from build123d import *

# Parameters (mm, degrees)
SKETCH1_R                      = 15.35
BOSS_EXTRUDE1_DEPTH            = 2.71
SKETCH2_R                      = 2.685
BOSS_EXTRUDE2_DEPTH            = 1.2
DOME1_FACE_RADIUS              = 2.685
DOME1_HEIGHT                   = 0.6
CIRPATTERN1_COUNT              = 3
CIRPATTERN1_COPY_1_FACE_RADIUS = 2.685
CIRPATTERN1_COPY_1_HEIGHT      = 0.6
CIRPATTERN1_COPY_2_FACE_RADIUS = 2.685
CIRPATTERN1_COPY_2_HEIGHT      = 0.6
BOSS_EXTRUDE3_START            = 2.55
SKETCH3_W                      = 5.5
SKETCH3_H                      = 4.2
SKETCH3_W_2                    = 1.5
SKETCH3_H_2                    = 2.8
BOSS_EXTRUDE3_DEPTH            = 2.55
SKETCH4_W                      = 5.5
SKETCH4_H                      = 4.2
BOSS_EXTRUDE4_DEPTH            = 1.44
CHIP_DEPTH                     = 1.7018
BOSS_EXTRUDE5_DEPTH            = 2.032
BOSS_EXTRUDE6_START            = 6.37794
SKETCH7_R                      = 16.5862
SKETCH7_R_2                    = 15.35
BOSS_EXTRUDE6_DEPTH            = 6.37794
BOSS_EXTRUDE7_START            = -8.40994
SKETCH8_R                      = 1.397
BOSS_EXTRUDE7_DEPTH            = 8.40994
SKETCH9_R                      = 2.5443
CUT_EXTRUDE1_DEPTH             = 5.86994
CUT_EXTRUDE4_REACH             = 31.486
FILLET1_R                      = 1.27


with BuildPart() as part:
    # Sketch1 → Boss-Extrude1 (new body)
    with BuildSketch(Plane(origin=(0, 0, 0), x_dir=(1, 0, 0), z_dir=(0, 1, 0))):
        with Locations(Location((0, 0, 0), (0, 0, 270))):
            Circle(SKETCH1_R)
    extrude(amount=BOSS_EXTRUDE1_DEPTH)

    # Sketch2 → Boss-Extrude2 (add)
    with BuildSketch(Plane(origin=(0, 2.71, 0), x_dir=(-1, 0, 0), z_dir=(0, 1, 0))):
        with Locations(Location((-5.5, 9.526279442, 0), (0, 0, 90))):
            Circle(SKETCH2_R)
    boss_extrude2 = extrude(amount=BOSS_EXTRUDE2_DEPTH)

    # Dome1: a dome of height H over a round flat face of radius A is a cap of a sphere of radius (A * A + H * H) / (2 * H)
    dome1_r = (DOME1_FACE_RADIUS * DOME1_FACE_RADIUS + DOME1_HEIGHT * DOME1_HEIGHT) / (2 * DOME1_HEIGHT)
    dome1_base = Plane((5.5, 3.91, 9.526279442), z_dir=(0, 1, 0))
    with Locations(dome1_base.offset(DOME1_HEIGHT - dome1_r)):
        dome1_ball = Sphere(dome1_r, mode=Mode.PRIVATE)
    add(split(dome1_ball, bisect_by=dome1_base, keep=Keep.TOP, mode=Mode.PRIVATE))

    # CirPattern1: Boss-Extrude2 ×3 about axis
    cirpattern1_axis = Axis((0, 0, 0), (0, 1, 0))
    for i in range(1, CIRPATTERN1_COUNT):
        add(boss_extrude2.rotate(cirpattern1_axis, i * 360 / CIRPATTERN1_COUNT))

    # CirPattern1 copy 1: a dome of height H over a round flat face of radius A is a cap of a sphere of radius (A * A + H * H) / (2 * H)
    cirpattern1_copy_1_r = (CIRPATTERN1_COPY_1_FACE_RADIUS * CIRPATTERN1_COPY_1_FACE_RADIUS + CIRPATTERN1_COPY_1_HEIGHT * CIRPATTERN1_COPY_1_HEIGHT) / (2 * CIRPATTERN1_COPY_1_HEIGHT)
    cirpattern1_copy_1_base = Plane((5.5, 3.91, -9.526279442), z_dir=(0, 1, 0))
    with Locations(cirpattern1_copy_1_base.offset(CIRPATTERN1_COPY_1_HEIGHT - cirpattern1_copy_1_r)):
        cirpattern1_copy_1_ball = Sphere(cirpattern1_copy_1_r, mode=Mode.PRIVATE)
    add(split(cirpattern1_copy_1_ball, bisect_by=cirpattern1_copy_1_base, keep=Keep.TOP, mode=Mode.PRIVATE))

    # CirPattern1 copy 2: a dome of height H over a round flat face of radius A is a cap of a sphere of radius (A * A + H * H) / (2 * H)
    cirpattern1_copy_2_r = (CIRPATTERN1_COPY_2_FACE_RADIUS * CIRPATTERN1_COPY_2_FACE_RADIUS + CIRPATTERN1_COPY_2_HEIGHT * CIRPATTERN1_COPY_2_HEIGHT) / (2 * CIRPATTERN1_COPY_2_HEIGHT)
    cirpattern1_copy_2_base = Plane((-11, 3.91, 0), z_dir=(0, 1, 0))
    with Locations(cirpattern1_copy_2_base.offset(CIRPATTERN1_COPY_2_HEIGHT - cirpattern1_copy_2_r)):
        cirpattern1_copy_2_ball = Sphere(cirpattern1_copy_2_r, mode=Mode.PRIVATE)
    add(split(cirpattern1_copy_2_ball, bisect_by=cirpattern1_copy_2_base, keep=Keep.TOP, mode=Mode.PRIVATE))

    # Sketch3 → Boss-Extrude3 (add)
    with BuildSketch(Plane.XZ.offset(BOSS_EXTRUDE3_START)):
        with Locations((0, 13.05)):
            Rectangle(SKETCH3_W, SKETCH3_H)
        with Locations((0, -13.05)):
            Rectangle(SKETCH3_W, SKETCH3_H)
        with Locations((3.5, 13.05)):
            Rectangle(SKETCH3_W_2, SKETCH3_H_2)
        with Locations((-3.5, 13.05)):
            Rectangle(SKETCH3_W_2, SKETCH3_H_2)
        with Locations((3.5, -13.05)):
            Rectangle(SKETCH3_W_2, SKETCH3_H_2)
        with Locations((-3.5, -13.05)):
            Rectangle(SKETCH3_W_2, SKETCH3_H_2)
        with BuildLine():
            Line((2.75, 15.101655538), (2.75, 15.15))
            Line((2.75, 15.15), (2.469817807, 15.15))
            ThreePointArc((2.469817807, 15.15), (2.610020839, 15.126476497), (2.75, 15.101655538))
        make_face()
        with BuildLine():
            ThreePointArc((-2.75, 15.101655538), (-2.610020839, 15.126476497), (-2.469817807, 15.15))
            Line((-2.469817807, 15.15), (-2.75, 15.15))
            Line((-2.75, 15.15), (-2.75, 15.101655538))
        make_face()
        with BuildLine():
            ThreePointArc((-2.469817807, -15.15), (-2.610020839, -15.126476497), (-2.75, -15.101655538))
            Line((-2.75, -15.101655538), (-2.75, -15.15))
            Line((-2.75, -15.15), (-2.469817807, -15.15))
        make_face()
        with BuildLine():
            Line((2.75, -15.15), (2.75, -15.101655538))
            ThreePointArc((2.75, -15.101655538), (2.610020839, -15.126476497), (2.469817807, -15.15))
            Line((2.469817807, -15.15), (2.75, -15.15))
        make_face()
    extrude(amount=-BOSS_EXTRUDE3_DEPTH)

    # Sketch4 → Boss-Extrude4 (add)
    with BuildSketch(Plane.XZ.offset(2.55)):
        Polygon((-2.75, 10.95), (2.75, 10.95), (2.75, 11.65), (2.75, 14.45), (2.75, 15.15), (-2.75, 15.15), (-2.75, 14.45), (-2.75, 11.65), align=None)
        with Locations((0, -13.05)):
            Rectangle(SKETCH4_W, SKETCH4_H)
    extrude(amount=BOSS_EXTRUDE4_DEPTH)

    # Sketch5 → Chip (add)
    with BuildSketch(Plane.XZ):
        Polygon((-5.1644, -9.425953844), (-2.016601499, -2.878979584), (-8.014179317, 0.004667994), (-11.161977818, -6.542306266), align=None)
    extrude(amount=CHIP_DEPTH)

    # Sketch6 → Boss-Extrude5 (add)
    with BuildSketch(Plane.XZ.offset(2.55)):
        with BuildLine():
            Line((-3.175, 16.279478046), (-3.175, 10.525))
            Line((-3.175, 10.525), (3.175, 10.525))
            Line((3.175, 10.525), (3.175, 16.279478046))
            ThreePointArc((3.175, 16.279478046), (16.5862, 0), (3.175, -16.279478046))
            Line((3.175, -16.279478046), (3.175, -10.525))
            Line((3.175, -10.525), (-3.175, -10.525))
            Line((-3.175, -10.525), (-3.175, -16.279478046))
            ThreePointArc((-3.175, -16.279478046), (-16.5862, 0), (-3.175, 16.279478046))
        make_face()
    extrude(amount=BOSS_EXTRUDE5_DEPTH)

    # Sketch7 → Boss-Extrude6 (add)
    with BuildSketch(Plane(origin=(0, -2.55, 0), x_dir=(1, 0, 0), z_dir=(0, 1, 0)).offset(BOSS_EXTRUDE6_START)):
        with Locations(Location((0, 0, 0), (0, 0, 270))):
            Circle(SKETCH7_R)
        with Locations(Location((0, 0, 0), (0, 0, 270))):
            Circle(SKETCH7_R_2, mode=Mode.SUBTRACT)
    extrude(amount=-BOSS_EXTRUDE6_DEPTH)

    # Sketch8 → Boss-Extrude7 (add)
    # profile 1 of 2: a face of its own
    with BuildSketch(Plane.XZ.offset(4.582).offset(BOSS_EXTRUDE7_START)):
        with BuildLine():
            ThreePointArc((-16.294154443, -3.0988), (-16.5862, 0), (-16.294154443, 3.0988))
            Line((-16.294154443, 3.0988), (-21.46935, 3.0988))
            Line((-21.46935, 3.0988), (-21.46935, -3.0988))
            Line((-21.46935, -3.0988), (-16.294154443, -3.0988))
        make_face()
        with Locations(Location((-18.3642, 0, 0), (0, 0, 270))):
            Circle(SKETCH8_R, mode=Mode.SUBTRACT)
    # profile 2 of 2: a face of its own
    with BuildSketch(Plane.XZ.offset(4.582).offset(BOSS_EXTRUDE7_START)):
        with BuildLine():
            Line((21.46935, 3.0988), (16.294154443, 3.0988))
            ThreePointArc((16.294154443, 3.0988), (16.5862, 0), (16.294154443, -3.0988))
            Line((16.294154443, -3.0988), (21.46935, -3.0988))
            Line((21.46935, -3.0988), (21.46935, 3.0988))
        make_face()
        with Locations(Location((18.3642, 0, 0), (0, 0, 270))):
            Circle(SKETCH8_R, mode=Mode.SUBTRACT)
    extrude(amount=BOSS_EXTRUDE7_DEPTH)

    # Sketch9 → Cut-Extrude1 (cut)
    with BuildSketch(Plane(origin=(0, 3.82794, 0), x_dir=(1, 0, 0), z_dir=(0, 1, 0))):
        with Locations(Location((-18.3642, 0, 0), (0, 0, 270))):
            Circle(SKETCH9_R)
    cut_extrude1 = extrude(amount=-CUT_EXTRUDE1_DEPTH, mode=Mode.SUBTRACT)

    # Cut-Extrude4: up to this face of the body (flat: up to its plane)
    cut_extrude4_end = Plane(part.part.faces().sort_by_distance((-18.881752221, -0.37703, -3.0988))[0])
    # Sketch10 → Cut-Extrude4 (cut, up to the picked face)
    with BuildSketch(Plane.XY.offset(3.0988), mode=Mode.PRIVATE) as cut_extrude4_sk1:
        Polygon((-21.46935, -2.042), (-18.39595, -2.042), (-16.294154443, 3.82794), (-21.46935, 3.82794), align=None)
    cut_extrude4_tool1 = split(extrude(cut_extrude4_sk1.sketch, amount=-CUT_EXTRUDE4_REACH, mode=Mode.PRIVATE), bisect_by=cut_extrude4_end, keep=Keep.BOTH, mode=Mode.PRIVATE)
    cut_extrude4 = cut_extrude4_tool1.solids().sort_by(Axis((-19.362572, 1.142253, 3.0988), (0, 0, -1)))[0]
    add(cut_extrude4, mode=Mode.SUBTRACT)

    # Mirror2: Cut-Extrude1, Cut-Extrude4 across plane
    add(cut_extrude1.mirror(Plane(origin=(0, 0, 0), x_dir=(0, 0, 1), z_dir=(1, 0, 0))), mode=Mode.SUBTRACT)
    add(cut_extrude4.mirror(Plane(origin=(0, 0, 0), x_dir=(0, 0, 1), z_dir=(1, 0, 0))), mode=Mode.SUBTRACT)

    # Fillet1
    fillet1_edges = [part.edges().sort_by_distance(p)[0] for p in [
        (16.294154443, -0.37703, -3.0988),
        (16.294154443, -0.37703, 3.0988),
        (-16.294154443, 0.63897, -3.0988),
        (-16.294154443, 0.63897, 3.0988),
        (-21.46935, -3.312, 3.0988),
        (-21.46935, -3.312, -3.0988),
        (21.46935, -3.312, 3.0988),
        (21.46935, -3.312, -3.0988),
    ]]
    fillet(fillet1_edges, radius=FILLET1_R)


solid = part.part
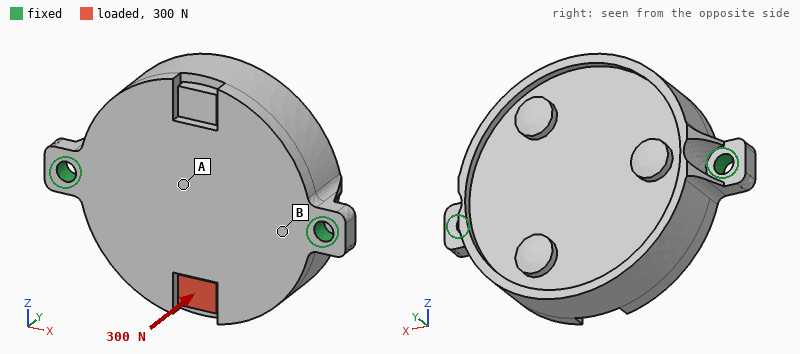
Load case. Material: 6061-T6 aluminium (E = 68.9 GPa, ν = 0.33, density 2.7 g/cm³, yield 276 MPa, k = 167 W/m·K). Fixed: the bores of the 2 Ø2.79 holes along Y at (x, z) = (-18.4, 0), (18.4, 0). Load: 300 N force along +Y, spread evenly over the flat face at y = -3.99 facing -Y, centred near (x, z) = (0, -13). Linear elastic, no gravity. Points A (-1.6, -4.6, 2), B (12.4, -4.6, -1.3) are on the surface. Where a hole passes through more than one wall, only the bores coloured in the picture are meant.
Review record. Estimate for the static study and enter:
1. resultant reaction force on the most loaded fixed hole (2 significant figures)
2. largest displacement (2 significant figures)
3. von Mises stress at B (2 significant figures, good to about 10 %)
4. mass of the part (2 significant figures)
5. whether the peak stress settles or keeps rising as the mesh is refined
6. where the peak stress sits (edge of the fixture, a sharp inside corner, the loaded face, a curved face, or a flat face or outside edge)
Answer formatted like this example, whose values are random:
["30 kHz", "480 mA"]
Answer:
["190 N", "95 µm", "32 MPa", "13 g", "keeps rising", "edge of the fixture"]
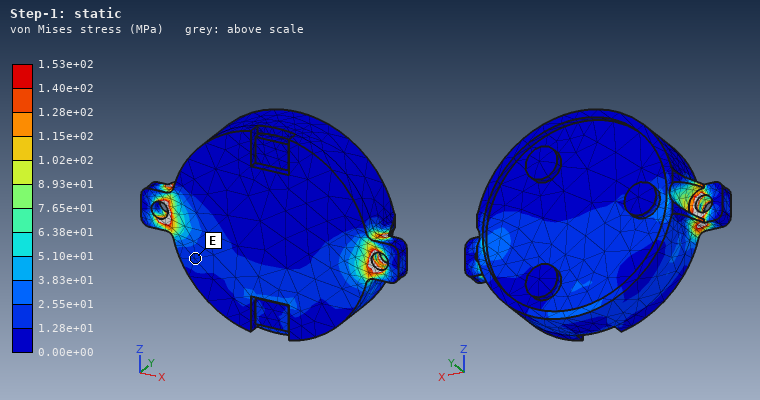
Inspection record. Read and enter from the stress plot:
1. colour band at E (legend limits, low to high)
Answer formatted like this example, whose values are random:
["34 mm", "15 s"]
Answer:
["1.28e+01 to 2.55e+01 MPa"]
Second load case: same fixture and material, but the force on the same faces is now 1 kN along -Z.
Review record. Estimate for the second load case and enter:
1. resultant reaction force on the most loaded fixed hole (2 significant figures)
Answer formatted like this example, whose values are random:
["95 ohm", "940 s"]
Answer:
["510 N"]
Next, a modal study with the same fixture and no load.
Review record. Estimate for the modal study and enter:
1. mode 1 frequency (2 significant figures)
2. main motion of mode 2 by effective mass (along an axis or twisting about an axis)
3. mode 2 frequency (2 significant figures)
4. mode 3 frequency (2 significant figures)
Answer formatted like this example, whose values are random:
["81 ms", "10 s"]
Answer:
["4400 Hz", "along Y", "9400 Hz", "18 kHz"]
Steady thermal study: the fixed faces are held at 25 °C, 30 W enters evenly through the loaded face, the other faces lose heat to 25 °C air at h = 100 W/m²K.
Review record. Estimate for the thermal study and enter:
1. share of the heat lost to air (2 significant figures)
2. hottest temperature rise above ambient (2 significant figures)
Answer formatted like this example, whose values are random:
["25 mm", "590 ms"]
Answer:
["29 %", "64 K"]
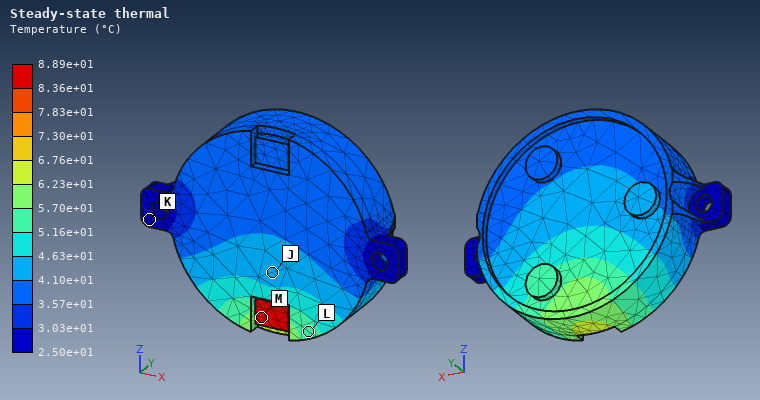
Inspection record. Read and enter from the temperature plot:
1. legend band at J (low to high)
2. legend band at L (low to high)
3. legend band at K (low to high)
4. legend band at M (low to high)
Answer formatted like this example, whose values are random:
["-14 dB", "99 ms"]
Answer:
["4.10e+01 to 4.63e+01 °C", "5.16e+01 to 5.70e+01 °C", "2.50e+01 to 3.03e+01 °C", "8.36e+01 to 8.89e+01 °C"]
